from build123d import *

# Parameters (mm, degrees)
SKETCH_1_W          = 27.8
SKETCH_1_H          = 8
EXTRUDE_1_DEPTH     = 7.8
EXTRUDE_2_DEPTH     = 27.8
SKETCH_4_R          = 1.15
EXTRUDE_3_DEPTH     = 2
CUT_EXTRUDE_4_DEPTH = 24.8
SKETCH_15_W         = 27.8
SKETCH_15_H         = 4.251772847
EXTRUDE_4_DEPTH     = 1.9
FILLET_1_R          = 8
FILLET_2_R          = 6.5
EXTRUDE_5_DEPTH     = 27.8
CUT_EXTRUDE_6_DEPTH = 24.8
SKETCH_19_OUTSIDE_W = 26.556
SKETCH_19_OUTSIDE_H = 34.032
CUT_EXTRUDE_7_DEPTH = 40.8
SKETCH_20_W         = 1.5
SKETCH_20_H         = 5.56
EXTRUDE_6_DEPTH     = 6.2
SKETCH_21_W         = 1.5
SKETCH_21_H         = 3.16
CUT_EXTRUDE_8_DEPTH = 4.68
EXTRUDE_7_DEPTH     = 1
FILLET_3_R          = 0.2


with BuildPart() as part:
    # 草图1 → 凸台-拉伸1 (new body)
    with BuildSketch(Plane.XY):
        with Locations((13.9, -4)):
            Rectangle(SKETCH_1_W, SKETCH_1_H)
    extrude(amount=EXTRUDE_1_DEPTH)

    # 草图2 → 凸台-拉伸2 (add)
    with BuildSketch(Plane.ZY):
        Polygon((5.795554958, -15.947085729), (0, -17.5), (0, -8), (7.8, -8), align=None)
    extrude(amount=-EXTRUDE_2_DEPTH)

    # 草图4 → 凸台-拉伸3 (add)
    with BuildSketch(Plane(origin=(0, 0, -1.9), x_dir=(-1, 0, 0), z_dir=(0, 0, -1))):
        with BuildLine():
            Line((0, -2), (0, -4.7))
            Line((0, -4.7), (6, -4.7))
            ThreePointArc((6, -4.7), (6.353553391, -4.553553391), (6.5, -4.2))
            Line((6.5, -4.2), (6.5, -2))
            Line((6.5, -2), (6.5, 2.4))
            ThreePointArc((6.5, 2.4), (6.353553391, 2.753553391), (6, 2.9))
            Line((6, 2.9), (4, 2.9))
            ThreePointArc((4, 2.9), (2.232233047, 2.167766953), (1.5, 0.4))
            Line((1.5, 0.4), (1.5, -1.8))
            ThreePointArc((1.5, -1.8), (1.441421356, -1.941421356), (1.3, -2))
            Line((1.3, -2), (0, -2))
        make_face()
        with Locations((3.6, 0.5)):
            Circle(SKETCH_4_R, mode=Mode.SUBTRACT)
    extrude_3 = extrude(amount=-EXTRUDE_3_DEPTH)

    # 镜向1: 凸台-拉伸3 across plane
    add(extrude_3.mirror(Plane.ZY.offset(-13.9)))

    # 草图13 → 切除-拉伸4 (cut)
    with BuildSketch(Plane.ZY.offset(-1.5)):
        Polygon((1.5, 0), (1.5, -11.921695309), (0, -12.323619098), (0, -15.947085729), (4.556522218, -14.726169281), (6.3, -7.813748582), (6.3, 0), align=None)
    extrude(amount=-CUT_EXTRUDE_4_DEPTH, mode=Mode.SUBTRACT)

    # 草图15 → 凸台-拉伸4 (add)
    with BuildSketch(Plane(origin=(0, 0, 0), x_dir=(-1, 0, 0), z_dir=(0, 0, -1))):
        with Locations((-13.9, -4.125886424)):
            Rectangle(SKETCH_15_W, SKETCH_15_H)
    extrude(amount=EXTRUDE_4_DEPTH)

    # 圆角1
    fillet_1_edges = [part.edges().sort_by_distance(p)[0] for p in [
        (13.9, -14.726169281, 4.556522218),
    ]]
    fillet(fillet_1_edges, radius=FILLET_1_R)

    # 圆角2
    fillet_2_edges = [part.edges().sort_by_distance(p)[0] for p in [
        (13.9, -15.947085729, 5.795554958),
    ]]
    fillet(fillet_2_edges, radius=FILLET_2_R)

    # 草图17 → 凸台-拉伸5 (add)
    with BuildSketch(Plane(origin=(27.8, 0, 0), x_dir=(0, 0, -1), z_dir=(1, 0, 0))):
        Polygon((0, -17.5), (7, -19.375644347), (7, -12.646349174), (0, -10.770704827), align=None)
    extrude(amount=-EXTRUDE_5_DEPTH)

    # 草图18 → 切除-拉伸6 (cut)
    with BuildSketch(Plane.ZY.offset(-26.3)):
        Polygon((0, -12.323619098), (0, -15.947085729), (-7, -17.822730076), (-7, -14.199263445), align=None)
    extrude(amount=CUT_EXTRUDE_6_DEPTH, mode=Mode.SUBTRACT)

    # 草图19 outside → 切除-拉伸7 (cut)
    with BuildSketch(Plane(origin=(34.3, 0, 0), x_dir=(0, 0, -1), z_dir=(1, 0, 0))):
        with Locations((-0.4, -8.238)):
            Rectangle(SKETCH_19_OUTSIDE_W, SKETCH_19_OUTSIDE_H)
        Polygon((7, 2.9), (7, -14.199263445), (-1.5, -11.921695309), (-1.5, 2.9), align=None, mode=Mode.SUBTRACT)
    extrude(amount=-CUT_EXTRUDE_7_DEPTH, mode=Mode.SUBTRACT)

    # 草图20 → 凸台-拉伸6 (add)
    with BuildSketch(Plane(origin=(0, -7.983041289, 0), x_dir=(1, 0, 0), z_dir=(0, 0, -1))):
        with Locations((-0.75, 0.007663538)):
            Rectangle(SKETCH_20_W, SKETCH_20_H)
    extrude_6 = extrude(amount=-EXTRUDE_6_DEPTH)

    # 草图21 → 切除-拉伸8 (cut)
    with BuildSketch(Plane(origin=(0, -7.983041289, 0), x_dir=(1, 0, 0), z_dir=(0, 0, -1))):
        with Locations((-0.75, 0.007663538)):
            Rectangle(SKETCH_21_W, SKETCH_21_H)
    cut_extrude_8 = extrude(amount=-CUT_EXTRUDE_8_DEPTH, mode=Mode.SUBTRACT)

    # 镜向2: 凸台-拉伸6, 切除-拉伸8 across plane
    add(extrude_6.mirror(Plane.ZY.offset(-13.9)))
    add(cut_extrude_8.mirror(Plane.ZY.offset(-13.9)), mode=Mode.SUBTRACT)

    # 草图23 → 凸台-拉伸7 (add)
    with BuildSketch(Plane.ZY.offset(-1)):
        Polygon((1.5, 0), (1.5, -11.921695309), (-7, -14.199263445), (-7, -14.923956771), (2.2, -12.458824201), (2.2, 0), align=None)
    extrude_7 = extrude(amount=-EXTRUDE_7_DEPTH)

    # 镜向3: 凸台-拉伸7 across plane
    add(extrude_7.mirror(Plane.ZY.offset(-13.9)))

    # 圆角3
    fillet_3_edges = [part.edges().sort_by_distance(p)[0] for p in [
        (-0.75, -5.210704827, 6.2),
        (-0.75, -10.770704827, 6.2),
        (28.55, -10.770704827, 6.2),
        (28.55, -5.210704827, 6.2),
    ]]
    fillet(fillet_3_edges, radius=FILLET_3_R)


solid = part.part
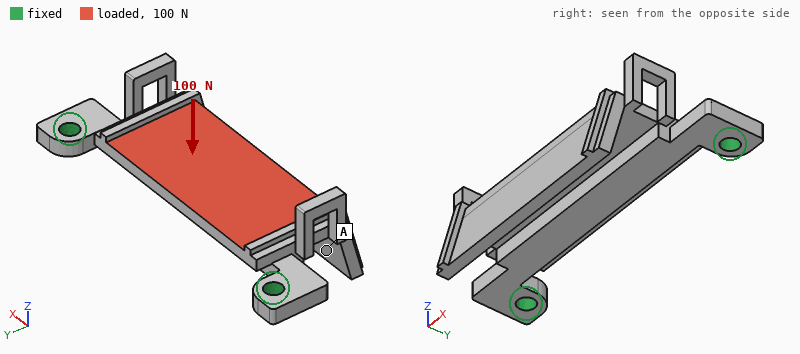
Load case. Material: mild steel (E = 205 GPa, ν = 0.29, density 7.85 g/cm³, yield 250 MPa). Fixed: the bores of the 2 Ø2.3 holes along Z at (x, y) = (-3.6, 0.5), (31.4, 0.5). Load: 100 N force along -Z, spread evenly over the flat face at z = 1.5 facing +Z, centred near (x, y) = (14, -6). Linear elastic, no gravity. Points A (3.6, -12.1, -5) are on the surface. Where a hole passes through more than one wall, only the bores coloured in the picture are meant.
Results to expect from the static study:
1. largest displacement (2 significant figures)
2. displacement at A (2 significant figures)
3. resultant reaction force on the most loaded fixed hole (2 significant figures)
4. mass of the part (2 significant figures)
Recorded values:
39 µm
30 µm
61 N
9.9 g
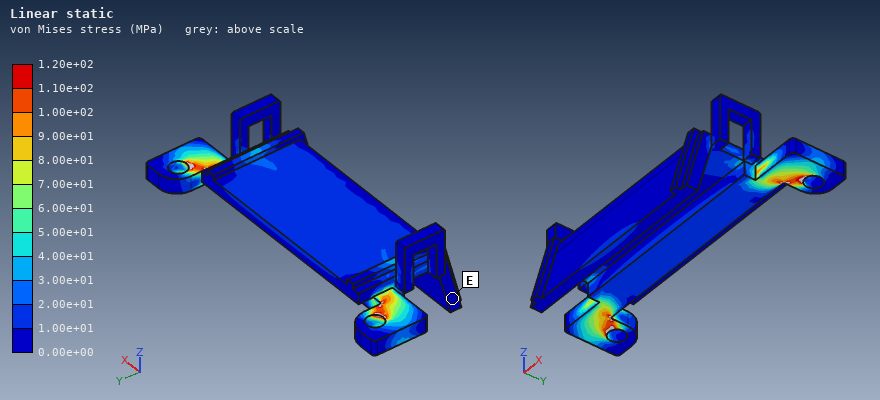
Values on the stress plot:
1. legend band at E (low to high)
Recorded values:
0.00e+00 to 1.00e+01 MPa
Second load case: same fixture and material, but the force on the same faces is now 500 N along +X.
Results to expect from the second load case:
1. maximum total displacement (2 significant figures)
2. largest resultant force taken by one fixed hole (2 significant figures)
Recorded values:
4.6 µm
260 N
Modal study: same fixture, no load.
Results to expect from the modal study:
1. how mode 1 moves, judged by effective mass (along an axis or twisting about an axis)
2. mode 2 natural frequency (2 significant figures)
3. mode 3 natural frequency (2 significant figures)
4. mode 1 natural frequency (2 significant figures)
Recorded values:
along Z
8000 Hz
8900 Hz
2700 Hz
